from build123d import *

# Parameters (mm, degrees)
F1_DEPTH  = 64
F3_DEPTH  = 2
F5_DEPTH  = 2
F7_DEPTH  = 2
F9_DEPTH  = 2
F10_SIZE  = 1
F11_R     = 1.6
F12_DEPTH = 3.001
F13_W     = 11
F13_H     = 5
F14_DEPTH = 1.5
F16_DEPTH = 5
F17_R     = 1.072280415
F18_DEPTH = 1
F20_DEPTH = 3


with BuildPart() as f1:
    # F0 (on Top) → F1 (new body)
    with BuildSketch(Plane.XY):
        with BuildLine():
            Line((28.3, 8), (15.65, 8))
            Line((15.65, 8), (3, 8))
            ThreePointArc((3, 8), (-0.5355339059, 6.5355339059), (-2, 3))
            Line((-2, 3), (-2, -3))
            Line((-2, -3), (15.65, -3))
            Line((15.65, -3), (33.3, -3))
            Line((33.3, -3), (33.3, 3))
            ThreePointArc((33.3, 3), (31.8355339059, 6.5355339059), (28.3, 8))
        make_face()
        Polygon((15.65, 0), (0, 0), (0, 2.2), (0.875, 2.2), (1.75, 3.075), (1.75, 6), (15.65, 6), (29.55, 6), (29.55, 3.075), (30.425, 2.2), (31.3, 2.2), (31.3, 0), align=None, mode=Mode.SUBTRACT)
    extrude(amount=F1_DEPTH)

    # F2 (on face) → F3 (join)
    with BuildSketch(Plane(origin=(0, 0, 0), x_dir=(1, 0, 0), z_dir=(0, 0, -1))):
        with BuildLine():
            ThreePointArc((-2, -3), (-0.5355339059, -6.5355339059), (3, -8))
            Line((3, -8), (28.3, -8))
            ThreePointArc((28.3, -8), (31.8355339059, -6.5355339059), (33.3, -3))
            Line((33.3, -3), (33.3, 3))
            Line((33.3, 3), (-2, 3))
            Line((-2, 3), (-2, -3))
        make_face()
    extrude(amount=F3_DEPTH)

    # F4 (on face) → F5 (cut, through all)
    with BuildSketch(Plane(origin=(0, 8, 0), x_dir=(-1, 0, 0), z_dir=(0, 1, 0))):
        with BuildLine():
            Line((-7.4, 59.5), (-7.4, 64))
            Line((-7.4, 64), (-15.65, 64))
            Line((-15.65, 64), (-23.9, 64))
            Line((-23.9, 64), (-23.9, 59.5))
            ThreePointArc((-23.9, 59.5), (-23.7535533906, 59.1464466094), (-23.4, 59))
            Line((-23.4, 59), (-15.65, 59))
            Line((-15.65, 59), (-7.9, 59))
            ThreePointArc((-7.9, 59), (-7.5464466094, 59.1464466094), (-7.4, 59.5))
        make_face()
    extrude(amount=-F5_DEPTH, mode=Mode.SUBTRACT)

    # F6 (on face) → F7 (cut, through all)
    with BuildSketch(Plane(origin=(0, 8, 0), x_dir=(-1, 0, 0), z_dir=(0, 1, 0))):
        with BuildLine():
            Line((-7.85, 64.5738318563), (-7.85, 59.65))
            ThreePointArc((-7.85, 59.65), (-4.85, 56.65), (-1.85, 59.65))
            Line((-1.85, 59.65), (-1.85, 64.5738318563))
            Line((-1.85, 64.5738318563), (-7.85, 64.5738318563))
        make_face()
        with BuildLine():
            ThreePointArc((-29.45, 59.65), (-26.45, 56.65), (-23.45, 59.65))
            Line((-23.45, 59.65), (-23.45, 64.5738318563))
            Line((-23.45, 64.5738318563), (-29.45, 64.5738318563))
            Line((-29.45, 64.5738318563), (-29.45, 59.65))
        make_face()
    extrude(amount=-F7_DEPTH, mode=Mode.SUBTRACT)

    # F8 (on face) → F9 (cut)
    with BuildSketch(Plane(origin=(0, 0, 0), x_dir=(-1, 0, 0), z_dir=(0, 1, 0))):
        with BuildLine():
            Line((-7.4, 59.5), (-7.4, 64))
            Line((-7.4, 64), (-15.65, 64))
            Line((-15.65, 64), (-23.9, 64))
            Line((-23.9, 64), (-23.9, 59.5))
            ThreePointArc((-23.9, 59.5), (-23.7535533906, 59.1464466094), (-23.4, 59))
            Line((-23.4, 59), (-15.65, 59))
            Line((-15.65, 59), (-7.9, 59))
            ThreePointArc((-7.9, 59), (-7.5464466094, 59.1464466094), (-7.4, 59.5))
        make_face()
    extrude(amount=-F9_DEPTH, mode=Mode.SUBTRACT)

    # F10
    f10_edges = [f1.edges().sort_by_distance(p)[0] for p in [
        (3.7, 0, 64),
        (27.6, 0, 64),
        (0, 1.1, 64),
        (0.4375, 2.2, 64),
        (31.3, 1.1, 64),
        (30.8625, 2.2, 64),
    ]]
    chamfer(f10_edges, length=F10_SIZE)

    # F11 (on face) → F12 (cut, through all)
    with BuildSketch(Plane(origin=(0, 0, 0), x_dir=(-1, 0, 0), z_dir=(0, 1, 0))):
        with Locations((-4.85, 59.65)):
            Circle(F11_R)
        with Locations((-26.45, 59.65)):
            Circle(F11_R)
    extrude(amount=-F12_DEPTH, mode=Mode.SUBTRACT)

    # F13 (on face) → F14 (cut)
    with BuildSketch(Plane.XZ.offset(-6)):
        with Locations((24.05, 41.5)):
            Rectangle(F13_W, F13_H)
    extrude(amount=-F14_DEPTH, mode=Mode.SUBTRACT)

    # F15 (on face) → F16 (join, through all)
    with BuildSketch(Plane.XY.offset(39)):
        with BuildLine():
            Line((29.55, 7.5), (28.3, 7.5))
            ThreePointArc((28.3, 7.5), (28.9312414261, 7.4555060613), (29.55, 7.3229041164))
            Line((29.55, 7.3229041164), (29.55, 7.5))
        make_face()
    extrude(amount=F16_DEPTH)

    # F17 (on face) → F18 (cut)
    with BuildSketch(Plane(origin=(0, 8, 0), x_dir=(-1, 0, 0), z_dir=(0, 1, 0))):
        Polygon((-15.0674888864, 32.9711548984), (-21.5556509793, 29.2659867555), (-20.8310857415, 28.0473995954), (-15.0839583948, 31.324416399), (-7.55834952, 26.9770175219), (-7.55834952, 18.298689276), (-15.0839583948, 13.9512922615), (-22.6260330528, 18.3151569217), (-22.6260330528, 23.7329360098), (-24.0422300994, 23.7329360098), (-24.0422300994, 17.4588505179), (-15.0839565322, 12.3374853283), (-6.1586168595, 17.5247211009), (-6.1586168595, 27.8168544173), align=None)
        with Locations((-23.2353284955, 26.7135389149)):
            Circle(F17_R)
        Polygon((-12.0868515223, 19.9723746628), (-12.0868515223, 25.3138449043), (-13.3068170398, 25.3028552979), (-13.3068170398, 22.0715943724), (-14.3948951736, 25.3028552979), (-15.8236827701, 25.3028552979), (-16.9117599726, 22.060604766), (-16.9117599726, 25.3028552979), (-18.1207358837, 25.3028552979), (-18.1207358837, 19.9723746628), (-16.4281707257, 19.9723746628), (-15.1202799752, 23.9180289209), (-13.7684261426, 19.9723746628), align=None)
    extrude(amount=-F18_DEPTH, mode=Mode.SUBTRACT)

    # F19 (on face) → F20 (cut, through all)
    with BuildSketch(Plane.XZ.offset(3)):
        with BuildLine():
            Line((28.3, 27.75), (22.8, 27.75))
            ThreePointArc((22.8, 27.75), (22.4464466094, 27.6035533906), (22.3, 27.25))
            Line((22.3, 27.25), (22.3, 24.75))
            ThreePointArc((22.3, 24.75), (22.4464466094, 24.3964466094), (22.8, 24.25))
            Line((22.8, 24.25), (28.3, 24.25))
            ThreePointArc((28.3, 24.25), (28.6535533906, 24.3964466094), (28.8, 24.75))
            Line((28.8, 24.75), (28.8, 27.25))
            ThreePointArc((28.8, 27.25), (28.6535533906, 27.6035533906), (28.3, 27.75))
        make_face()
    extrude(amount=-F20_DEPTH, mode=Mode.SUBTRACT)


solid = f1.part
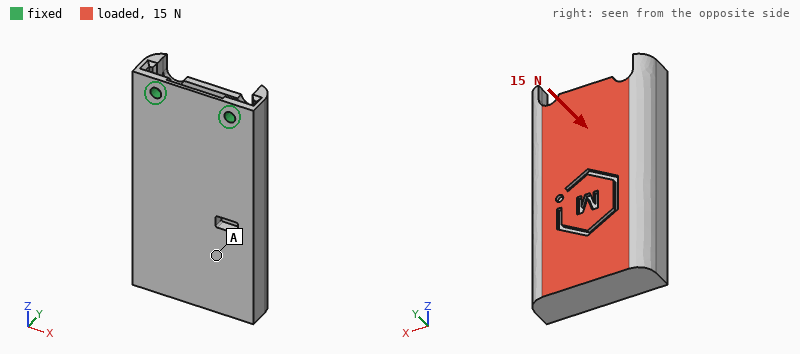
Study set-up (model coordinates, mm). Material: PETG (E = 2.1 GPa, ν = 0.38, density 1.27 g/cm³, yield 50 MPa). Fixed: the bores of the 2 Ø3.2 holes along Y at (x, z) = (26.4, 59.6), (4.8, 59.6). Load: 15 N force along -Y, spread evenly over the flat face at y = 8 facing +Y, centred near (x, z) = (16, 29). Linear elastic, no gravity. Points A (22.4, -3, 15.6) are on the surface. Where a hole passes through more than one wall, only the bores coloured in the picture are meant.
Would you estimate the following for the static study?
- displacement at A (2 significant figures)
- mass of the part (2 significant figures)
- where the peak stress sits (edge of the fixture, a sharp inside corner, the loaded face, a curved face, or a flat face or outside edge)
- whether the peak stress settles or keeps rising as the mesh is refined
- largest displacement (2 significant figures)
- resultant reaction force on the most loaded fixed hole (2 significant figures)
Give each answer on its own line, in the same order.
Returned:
0.59 mm
16 g
edge of the fixture
keeps rising
0.85 mm
8.3 N
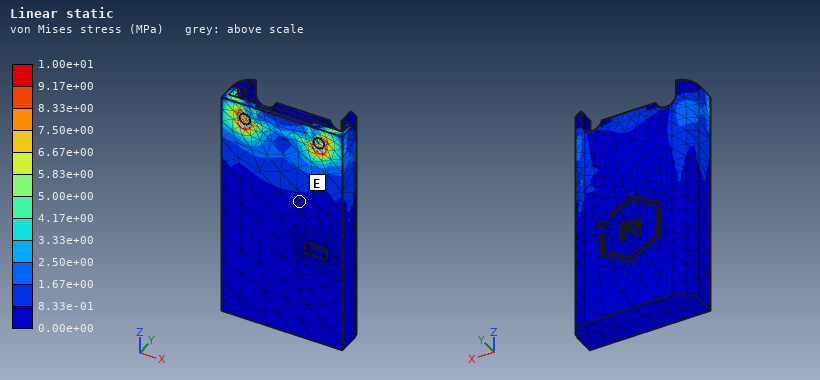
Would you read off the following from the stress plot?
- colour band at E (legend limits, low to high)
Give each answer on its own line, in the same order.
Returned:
0.00e+00 to 8.33e-01 MPa
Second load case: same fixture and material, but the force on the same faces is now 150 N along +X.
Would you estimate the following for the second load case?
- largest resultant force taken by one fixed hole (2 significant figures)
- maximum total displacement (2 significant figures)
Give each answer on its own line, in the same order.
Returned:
210 N
0.51 mm
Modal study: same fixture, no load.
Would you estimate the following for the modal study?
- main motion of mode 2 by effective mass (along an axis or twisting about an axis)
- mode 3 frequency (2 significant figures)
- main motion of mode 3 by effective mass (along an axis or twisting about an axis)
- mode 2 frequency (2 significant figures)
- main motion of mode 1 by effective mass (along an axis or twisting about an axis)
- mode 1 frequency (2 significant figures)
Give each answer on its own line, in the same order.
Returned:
along X
1000 Hz
along X
990 Hz
along Y
200 Hz
